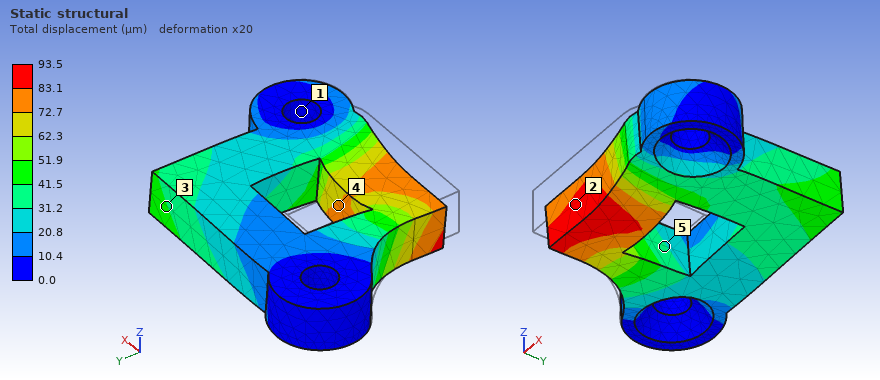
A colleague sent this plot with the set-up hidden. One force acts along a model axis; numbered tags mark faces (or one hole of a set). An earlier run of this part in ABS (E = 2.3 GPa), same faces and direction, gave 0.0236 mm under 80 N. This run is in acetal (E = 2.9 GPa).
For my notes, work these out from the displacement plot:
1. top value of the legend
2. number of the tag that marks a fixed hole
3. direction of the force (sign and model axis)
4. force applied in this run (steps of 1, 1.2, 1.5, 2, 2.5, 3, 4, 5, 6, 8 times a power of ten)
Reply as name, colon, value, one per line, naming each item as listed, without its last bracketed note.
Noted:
top value of the legend: 93.5 µm
number of the tag that marks a fixed hole: 1
direction of the force: +Y
force applied in this run: 400 N
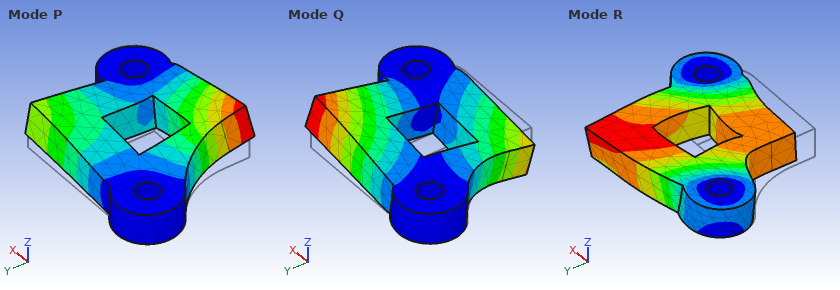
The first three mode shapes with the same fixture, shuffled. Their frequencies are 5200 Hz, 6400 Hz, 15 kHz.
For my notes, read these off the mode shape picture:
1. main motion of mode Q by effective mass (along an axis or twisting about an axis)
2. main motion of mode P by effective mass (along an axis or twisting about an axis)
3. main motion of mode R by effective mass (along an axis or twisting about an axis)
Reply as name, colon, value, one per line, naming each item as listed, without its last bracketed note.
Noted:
main motion of mode Q by effective mass: twisting about X
main motion of mode P by effective mass: along Z
main motion of mode R by effective mass: along Y
